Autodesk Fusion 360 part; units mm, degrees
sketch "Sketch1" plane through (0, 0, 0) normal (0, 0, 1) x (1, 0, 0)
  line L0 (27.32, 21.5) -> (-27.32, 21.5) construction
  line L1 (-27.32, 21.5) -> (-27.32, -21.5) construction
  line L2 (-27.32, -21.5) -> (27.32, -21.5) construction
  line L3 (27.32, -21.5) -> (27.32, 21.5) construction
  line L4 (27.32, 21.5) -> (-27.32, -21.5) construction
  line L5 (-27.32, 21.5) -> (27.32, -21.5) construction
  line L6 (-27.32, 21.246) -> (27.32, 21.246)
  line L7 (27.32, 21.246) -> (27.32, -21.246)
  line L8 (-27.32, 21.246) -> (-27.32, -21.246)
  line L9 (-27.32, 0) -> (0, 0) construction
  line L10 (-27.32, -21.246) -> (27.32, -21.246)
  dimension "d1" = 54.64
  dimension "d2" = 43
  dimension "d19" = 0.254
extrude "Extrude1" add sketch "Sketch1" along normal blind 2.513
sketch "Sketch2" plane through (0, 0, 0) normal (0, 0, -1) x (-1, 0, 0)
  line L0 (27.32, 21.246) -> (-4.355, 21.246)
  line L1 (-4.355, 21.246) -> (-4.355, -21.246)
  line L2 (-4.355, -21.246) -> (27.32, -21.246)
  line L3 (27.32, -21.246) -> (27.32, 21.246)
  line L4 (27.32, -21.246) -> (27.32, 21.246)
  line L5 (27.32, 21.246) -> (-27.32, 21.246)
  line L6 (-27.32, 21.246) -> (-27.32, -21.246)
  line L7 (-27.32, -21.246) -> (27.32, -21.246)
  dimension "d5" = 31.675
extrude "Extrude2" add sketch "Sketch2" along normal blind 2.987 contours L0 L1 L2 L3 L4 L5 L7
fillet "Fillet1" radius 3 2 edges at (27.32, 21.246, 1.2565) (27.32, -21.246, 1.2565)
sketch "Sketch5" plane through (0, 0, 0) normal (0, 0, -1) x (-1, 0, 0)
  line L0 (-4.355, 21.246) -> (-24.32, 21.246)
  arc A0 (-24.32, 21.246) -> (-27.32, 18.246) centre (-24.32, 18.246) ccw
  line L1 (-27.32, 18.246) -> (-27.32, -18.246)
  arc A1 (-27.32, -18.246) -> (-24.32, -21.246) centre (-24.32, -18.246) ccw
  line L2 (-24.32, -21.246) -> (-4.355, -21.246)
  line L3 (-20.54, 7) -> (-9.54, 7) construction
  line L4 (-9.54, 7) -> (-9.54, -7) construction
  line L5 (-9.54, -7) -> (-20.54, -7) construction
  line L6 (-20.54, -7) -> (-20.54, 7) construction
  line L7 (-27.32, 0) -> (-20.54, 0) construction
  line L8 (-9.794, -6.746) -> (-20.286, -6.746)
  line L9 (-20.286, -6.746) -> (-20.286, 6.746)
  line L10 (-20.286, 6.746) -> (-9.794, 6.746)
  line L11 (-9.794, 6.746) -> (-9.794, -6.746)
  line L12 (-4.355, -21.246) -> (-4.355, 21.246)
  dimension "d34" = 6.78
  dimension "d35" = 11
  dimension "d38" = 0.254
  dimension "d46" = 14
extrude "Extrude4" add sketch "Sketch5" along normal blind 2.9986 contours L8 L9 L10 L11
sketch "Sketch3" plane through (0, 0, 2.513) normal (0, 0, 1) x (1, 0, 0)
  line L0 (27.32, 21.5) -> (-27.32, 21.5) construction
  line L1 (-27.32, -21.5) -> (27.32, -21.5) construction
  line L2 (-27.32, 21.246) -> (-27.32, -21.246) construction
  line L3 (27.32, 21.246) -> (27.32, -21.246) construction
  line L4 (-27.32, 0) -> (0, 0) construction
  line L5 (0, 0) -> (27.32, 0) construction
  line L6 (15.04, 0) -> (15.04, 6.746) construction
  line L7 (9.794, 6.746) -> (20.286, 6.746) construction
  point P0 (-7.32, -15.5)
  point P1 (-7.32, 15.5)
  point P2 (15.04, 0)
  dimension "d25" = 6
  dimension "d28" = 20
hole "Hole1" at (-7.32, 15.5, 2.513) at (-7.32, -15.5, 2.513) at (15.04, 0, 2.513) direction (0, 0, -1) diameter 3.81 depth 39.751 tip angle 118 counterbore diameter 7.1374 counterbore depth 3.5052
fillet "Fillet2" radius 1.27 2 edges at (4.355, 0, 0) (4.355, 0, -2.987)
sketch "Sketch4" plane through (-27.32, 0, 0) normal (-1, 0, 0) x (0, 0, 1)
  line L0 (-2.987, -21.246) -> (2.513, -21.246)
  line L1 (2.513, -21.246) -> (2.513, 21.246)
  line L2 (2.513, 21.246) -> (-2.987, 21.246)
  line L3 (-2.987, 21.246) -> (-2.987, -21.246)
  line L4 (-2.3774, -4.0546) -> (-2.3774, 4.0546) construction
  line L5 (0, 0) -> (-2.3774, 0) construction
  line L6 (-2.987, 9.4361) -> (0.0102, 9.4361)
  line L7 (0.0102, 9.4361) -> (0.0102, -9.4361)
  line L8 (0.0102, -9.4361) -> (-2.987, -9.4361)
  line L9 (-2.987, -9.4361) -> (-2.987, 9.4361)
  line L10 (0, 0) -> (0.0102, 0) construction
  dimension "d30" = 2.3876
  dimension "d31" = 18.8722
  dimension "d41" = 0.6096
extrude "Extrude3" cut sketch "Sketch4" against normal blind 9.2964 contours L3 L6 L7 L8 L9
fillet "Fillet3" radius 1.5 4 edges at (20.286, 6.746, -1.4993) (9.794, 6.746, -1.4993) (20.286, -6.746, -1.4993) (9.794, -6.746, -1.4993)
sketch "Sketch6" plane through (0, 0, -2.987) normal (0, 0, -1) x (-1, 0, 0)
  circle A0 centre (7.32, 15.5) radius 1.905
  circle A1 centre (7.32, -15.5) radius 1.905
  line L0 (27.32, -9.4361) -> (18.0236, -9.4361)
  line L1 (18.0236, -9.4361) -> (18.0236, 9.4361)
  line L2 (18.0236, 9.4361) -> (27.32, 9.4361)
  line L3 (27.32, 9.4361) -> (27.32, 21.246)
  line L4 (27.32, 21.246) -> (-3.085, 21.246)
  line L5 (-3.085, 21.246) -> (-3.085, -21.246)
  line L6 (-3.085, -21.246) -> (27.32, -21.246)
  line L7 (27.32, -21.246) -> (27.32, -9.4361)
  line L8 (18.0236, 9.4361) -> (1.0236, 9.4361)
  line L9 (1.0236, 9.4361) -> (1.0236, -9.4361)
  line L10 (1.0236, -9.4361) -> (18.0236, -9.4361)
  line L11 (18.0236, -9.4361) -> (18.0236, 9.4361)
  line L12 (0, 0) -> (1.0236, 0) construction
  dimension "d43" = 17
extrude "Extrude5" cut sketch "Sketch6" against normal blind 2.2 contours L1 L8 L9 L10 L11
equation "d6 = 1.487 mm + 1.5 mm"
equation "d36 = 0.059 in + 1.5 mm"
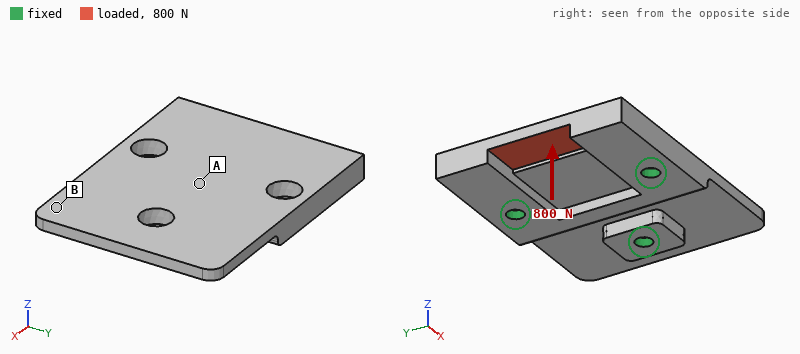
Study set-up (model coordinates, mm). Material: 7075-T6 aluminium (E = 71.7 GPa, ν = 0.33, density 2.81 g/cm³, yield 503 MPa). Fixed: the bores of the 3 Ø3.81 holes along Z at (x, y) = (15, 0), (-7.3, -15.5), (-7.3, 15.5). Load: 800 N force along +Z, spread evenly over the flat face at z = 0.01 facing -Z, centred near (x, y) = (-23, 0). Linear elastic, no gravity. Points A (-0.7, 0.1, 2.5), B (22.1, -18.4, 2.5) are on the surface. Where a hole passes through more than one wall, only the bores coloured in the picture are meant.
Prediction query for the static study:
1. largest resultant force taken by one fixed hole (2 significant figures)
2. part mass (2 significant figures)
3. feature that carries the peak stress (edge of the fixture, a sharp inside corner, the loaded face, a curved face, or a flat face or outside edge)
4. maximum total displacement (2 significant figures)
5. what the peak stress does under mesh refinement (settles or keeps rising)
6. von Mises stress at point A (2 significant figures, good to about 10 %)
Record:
1.0 kN
24 g
edge of the fixture
0.15 mm
keeps rising
47 MPa
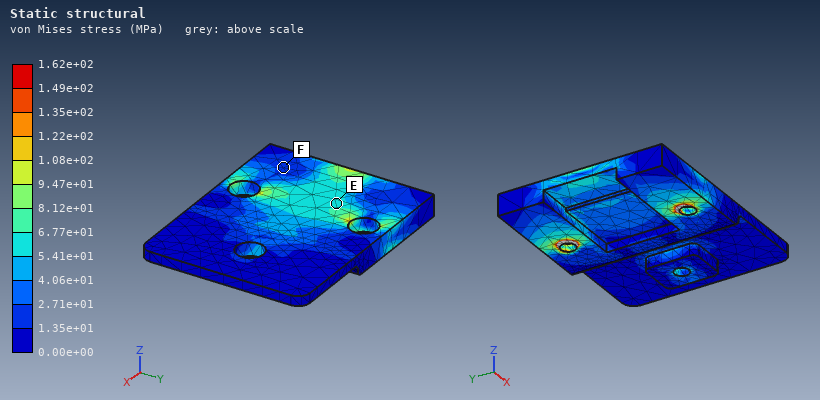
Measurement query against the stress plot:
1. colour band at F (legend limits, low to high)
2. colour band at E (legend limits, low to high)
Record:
1.35e+01 to 2.71e+01 MPa
5.41e+01 to 6.77e+01 MPa
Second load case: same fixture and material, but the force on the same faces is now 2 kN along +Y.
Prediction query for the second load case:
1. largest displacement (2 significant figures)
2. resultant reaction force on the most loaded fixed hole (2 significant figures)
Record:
42 µm
1.3 kN
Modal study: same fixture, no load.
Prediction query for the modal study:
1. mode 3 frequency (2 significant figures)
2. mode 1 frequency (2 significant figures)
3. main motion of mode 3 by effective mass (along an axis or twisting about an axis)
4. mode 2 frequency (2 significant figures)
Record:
8800 Hz
6700 Hz
along Z
7500 Hz
